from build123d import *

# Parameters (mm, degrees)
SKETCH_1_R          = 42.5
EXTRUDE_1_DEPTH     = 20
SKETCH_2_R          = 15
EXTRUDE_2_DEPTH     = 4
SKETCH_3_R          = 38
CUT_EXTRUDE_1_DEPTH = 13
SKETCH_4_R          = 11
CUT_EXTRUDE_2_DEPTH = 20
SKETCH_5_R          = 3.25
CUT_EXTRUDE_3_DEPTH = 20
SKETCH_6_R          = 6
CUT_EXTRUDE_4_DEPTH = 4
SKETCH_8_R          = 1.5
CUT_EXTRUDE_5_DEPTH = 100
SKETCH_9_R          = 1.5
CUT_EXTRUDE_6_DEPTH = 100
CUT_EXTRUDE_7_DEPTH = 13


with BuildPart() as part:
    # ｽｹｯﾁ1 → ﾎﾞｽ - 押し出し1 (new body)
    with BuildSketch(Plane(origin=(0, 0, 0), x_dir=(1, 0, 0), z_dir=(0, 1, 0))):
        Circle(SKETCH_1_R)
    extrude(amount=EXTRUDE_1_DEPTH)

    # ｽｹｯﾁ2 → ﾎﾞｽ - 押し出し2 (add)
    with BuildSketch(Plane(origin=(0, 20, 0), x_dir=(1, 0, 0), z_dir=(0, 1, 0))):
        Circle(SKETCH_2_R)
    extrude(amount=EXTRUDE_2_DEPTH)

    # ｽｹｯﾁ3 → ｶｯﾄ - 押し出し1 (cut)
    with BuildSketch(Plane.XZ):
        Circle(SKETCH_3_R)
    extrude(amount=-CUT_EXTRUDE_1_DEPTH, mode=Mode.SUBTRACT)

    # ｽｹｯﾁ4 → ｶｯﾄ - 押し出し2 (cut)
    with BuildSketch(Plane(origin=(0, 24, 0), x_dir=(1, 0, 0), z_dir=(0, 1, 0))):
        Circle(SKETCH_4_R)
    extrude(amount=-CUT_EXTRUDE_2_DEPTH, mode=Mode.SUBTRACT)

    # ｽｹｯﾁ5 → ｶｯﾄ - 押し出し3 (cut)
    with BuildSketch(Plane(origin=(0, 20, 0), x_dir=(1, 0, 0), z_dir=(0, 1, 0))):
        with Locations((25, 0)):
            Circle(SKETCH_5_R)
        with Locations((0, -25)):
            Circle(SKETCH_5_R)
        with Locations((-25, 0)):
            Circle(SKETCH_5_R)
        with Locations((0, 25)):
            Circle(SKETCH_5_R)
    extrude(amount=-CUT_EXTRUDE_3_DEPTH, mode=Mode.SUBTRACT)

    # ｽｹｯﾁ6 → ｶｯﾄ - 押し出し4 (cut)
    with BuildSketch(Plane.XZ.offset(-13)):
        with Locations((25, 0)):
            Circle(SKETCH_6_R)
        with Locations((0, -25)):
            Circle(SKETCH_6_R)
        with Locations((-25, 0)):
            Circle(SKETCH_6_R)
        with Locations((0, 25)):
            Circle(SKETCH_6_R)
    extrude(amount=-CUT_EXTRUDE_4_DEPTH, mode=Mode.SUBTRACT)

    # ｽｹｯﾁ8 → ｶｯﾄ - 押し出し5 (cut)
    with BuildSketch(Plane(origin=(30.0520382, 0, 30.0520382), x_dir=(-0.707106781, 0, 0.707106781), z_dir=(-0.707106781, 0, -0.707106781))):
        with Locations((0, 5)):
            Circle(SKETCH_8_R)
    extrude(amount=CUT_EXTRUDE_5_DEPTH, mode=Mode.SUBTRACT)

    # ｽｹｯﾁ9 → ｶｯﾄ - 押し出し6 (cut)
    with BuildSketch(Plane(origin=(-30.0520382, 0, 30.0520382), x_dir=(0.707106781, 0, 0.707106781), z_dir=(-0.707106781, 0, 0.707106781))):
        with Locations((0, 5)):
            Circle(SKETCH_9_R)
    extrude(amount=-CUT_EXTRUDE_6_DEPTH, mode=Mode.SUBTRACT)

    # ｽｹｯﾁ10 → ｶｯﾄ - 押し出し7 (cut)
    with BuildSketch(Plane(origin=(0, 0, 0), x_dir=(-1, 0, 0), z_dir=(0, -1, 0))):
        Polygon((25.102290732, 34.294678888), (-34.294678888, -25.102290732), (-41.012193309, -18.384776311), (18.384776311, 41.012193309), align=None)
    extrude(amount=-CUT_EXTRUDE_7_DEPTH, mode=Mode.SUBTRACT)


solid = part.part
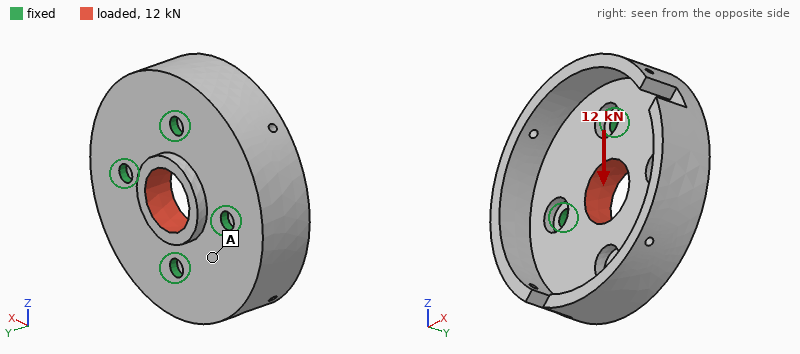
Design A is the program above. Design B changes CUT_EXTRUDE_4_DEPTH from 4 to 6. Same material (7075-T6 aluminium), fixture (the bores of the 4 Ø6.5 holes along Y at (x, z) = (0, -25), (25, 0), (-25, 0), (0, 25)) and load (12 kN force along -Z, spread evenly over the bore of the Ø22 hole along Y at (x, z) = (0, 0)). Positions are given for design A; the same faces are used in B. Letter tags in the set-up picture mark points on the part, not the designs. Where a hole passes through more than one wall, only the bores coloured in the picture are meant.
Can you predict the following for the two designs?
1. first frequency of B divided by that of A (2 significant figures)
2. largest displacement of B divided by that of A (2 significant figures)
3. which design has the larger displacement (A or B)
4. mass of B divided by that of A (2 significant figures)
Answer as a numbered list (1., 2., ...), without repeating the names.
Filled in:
1. 0.81
2. 2.2
3. B
4. 0.99
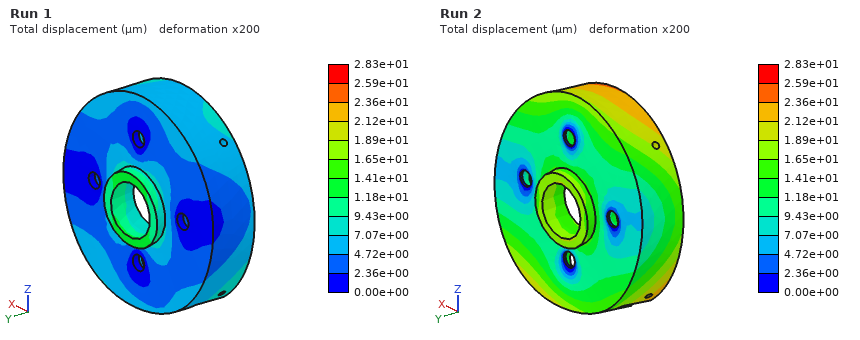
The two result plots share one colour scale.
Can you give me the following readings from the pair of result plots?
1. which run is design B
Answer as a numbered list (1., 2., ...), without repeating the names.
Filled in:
1. Run 2
